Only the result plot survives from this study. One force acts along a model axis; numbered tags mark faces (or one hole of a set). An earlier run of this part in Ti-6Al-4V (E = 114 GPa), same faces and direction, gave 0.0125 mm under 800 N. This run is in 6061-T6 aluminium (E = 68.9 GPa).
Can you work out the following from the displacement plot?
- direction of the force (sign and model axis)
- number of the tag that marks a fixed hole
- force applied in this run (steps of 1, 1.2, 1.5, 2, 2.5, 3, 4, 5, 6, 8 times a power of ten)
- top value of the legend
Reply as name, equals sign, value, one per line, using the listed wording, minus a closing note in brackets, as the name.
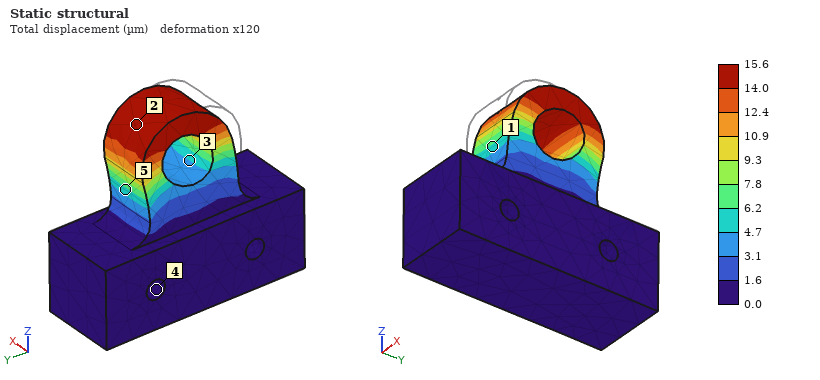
direction of the force = +Y
number of the tag that marks a fixed hole = 4
force applied in this run = 600 N
top value of the legend = 15.6 µm
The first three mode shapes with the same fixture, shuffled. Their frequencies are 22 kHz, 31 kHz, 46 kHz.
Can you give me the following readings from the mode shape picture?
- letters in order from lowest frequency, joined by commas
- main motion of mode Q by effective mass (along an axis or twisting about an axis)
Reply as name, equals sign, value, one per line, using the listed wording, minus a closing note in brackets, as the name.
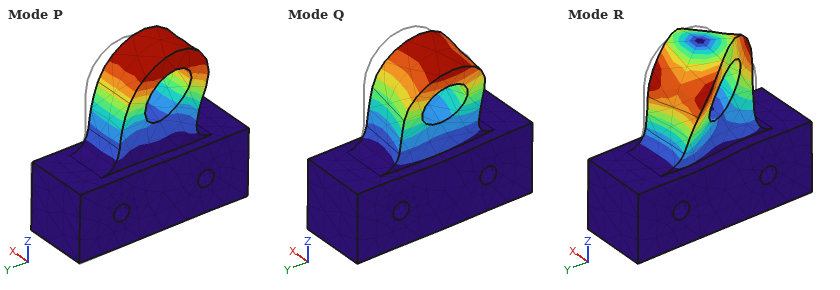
letters in order from lowest frequency, joined by commas = Q, P, R
main motion of mode Q by effective mass = along X
